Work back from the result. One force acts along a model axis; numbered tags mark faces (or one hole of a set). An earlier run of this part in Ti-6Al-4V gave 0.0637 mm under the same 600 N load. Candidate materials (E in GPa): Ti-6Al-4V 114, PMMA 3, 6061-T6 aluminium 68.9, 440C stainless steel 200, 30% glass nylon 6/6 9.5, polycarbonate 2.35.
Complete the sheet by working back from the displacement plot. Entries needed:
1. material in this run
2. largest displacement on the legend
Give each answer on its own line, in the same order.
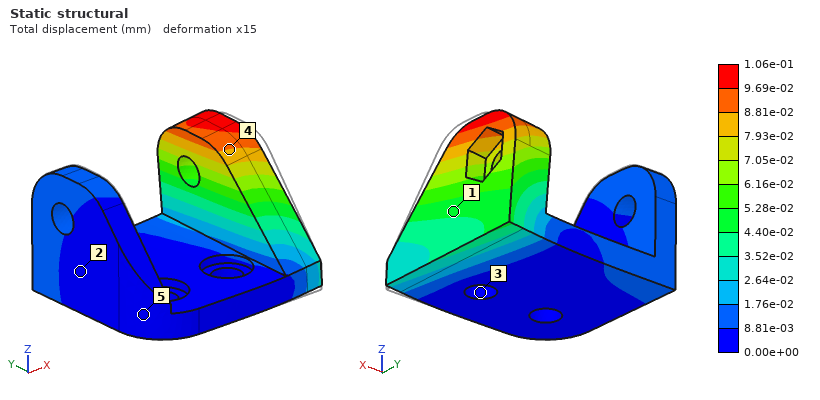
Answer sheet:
6061-T6 aluminium
1.06e-01 mm
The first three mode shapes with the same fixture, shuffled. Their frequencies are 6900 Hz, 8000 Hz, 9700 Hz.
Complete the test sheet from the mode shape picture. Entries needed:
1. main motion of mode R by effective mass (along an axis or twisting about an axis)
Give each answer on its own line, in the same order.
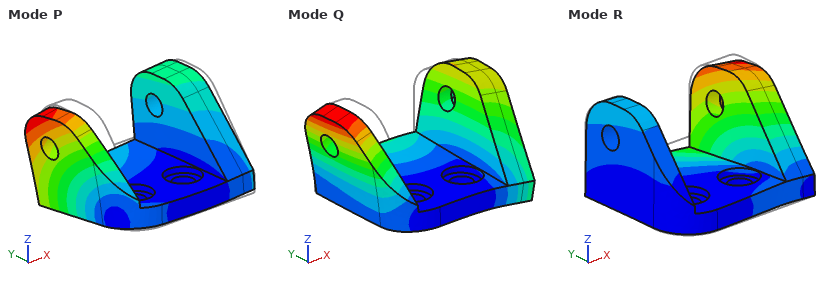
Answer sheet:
along Z
